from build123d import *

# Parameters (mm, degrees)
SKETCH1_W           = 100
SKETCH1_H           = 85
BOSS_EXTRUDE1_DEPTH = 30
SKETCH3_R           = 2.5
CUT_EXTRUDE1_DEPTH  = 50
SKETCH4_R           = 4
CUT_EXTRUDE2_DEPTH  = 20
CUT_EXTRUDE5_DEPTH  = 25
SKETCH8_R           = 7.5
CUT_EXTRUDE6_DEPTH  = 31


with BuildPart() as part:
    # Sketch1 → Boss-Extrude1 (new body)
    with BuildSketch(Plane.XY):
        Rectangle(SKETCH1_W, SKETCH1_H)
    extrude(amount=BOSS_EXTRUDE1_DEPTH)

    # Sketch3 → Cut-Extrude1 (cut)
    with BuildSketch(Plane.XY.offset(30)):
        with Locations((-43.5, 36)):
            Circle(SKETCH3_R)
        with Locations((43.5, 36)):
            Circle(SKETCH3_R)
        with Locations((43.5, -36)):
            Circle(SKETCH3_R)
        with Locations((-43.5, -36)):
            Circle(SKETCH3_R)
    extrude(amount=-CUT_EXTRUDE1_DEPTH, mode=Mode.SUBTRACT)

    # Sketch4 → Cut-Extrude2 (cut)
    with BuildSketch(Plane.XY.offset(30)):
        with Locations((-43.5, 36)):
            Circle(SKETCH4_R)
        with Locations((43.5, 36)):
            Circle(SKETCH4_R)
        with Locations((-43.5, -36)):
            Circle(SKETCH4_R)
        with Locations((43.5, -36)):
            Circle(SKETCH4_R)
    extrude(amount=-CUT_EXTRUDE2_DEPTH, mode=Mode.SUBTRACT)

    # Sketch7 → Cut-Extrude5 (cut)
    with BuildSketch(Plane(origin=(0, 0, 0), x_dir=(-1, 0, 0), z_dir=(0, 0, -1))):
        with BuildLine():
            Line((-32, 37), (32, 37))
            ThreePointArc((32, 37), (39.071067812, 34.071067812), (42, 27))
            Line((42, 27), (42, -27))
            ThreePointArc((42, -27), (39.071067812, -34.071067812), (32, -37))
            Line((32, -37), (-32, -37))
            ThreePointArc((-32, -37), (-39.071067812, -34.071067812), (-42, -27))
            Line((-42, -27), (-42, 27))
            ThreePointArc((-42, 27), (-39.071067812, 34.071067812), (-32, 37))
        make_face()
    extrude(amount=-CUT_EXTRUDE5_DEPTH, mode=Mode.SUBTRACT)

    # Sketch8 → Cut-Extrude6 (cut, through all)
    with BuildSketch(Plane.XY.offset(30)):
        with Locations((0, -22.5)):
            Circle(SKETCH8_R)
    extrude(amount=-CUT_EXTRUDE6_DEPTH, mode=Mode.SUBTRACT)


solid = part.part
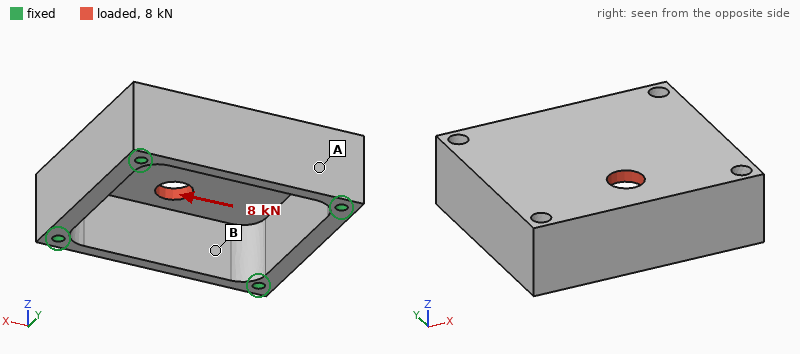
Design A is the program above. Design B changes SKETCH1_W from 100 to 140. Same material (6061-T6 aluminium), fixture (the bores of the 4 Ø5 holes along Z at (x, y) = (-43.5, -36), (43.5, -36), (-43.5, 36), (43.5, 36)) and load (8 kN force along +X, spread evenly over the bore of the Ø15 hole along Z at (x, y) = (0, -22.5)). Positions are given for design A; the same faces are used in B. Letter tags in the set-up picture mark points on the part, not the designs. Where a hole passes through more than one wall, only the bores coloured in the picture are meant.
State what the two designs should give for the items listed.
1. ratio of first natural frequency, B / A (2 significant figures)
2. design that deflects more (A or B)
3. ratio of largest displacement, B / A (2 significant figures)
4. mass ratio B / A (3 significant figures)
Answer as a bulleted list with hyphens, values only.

- 1.0
- A
- 0.89
- 2.06
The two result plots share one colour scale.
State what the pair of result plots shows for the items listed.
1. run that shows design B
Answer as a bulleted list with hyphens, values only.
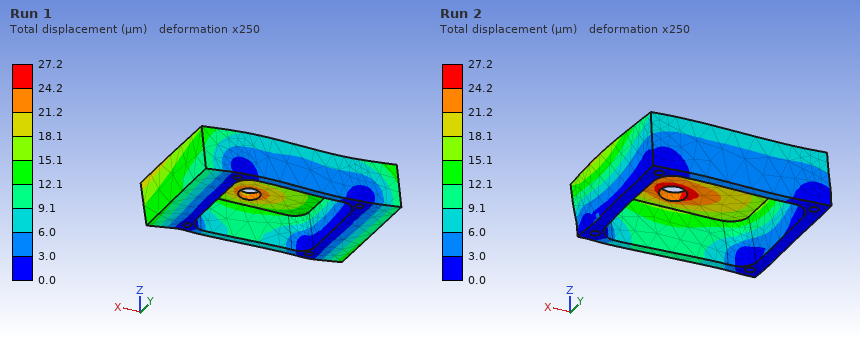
- Run 1
